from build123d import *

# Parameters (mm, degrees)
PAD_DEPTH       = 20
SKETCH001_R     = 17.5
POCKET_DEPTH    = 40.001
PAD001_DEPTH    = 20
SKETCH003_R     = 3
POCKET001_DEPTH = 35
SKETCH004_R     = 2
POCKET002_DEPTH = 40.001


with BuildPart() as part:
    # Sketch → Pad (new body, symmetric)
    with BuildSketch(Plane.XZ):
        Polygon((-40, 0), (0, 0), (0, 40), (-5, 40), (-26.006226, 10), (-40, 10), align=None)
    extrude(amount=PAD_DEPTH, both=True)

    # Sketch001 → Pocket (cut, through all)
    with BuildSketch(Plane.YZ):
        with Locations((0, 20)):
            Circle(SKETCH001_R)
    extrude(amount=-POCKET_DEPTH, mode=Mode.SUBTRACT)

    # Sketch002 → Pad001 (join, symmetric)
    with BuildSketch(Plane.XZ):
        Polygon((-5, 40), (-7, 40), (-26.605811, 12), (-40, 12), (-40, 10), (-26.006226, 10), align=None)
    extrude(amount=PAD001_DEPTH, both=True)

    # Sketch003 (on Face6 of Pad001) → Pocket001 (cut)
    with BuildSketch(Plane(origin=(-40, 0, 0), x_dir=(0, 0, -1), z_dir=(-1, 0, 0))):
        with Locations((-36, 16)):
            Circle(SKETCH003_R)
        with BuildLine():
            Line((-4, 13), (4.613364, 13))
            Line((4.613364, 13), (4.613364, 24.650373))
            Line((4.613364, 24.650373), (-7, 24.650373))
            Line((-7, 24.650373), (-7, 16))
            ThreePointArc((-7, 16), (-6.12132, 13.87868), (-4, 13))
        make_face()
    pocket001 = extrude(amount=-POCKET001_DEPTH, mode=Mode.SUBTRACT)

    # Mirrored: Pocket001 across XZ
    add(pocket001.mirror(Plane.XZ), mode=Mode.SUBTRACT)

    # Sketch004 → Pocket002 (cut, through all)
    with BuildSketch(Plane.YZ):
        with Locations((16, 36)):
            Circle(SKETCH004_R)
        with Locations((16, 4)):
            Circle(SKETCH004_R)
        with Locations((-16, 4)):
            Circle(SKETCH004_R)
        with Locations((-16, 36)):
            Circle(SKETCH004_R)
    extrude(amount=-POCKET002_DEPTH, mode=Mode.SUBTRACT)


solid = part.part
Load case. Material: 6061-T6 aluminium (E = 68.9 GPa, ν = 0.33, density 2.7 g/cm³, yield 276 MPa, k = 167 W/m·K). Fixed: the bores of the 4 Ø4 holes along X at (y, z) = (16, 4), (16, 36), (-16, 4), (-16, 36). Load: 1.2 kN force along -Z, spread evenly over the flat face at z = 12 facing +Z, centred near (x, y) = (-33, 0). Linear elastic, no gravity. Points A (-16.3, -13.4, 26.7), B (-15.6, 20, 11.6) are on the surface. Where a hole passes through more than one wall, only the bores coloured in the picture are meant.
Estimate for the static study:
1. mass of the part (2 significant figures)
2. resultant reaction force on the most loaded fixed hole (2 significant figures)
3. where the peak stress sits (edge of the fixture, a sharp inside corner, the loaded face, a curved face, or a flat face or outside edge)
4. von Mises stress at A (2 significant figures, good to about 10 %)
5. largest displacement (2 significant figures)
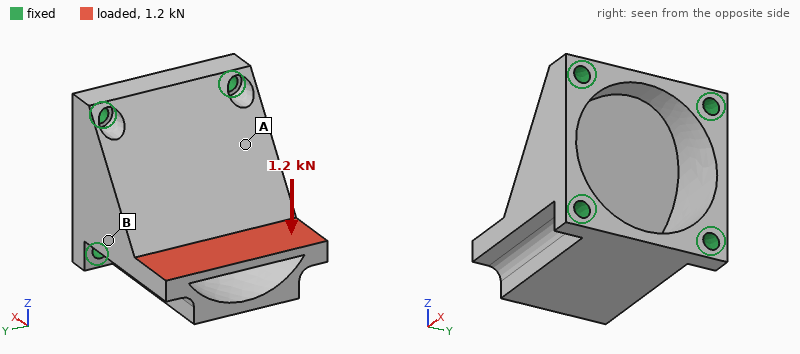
38 g
760 N
the loaded face
18 MPa
0.14 mm
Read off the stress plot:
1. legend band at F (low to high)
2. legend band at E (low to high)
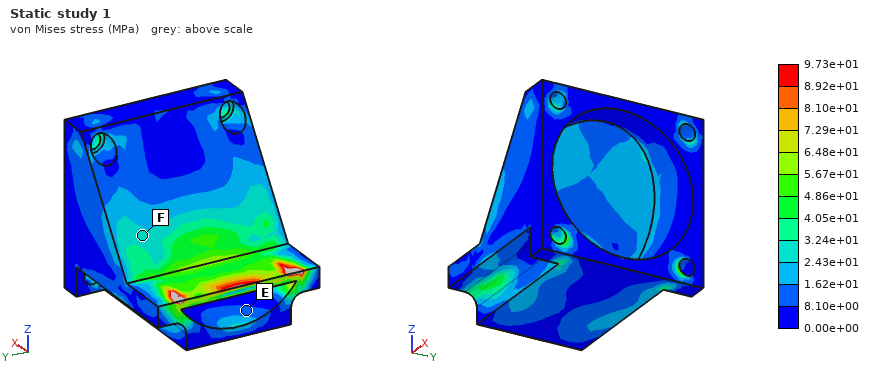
2.43e+01 to 3.24e+01 MPa
8.10e+00 to 1.62e+01 MPa
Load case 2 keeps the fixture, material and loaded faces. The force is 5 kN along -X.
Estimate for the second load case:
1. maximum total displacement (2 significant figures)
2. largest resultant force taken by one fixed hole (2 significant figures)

0.12 mm
2.0 kN
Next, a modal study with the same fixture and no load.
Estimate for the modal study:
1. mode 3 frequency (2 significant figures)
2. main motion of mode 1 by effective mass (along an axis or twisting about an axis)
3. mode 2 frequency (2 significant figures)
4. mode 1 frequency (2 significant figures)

11 kHz
along Z
11 kHz
9500 Hz
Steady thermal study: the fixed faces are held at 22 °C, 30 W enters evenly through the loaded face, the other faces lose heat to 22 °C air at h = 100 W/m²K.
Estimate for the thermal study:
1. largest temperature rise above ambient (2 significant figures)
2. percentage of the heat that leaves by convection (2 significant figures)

31 K
27 %
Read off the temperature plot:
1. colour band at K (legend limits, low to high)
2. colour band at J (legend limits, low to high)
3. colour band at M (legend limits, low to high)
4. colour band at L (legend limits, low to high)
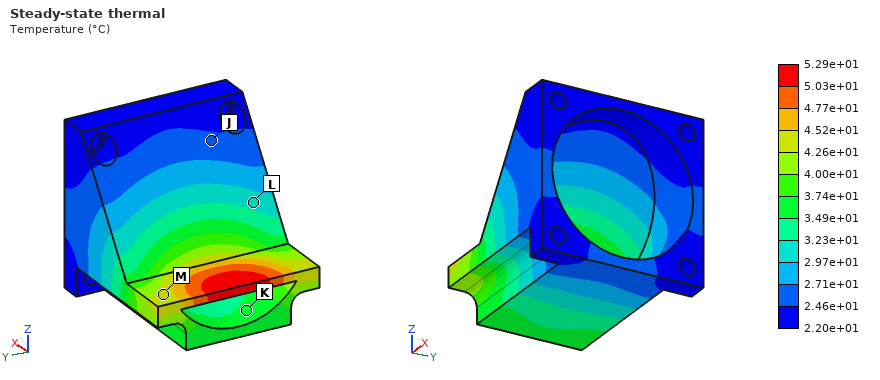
3.49e+01 to 3.74e+01 °C
2.46e+01 to 2.71e+01 °C
4.26e+01 to 4.52e+01 °C
2.97e+01 to 3.23e+01 °C
